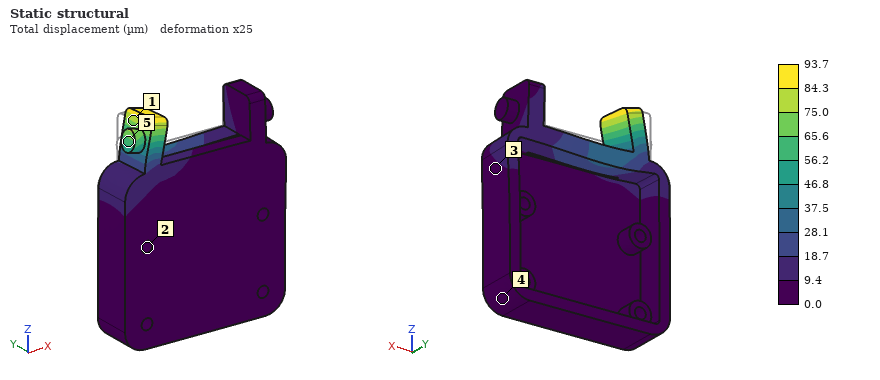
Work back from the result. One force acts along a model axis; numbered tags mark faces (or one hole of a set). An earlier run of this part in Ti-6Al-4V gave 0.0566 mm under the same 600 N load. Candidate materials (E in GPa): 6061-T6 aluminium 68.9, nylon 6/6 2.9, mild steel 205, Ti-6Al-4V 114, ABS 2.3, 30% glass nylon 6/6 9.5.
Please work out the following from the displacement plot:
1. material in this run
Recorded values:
6061-T6 aluminium
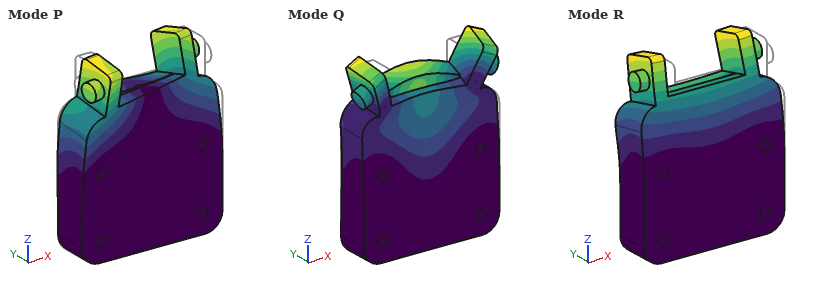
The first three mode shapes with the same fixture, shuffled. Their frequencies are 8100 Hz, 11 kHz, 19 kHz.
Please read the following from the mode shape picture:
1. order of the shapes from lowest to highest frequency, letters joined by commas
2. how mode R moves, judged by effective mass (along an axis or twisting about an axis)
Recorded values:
R, P, Q
along Y
